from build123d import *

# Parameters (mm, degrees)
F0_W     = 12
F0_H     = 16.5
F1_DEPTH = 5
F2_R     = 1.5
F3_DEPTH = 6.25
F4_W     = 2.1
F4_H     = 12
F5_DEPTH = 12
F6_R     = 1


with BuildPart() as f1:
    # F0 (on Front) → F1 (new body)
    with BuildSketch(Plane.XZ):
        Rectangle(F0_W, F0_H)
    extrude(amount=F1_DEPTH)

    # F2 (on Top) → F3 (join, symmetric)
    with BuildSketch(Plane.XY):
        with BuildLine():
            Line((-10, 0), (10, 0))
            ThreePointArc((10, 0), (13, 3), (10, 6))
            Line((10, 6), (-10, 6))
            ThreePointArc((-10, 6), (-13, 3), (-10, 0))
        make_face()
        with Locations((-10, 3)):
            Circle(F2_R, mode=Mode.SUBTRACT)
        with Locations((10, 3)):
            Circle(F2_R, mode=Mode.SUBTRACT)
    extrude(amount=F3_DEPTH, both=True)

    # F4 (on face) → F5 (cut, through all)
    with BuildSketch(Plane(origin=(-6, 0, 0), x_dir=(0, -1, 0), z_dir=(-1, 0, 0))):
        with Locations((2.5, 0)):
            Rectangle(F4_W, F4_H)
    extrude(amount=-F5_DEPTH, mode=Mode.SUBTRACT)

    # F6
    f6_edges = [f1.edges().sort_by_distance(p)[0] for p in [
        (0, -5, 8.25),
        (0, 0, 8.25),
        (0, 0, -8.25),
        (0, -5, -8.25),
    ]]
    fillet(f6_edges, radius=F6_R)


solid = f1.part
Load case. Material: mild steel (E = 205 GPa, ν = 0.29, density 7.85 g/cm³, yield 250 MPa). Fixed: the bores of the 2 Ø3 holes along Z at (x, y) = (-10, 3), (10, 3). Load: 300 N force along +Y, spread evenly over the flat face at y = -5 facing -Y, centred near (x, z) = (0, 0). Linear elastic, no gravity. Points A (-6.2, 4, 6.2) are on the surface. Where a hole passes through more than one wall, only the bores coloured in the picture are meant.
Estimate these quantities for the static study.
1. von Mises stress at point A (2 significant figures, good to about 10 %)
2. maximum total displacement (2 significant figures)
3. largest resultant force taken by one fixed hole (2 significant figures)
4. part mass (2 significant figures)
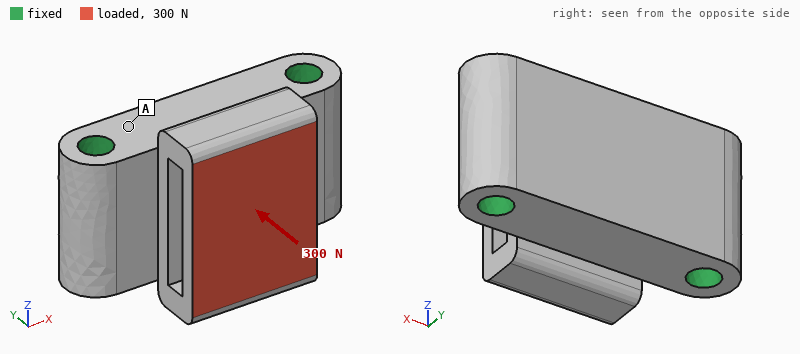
5.9 MPa
4.5 µm
160 N
18 g
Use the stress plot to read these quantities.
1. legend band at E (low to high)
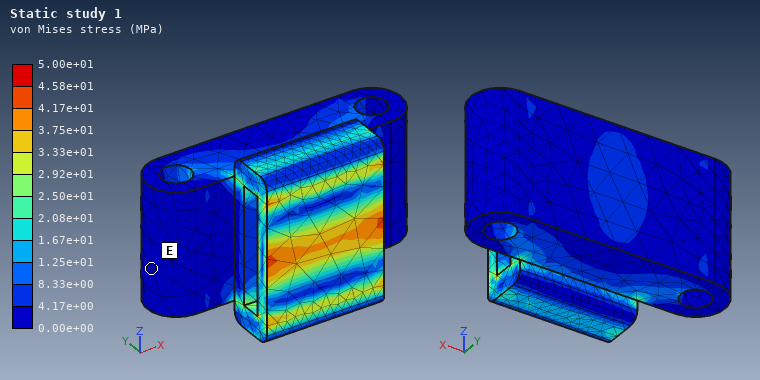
0.00e+00 to 4.17e+00 MPa
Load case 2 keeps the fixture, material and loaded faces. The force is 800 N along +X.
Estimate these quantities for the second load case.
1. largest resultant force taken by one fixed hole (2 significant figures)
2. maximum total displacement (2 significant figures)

550 N
6.2 µm
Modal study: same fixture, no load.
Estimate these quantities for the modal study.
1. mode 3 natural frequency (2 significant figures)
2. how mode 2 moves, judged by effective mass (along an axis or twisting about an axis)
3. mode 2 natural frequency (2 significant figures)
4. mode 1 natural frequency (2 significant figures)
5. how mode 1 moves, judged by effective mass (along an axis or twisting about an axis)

41 kHz
along Y
33 kHz
26 kHz
along Z
